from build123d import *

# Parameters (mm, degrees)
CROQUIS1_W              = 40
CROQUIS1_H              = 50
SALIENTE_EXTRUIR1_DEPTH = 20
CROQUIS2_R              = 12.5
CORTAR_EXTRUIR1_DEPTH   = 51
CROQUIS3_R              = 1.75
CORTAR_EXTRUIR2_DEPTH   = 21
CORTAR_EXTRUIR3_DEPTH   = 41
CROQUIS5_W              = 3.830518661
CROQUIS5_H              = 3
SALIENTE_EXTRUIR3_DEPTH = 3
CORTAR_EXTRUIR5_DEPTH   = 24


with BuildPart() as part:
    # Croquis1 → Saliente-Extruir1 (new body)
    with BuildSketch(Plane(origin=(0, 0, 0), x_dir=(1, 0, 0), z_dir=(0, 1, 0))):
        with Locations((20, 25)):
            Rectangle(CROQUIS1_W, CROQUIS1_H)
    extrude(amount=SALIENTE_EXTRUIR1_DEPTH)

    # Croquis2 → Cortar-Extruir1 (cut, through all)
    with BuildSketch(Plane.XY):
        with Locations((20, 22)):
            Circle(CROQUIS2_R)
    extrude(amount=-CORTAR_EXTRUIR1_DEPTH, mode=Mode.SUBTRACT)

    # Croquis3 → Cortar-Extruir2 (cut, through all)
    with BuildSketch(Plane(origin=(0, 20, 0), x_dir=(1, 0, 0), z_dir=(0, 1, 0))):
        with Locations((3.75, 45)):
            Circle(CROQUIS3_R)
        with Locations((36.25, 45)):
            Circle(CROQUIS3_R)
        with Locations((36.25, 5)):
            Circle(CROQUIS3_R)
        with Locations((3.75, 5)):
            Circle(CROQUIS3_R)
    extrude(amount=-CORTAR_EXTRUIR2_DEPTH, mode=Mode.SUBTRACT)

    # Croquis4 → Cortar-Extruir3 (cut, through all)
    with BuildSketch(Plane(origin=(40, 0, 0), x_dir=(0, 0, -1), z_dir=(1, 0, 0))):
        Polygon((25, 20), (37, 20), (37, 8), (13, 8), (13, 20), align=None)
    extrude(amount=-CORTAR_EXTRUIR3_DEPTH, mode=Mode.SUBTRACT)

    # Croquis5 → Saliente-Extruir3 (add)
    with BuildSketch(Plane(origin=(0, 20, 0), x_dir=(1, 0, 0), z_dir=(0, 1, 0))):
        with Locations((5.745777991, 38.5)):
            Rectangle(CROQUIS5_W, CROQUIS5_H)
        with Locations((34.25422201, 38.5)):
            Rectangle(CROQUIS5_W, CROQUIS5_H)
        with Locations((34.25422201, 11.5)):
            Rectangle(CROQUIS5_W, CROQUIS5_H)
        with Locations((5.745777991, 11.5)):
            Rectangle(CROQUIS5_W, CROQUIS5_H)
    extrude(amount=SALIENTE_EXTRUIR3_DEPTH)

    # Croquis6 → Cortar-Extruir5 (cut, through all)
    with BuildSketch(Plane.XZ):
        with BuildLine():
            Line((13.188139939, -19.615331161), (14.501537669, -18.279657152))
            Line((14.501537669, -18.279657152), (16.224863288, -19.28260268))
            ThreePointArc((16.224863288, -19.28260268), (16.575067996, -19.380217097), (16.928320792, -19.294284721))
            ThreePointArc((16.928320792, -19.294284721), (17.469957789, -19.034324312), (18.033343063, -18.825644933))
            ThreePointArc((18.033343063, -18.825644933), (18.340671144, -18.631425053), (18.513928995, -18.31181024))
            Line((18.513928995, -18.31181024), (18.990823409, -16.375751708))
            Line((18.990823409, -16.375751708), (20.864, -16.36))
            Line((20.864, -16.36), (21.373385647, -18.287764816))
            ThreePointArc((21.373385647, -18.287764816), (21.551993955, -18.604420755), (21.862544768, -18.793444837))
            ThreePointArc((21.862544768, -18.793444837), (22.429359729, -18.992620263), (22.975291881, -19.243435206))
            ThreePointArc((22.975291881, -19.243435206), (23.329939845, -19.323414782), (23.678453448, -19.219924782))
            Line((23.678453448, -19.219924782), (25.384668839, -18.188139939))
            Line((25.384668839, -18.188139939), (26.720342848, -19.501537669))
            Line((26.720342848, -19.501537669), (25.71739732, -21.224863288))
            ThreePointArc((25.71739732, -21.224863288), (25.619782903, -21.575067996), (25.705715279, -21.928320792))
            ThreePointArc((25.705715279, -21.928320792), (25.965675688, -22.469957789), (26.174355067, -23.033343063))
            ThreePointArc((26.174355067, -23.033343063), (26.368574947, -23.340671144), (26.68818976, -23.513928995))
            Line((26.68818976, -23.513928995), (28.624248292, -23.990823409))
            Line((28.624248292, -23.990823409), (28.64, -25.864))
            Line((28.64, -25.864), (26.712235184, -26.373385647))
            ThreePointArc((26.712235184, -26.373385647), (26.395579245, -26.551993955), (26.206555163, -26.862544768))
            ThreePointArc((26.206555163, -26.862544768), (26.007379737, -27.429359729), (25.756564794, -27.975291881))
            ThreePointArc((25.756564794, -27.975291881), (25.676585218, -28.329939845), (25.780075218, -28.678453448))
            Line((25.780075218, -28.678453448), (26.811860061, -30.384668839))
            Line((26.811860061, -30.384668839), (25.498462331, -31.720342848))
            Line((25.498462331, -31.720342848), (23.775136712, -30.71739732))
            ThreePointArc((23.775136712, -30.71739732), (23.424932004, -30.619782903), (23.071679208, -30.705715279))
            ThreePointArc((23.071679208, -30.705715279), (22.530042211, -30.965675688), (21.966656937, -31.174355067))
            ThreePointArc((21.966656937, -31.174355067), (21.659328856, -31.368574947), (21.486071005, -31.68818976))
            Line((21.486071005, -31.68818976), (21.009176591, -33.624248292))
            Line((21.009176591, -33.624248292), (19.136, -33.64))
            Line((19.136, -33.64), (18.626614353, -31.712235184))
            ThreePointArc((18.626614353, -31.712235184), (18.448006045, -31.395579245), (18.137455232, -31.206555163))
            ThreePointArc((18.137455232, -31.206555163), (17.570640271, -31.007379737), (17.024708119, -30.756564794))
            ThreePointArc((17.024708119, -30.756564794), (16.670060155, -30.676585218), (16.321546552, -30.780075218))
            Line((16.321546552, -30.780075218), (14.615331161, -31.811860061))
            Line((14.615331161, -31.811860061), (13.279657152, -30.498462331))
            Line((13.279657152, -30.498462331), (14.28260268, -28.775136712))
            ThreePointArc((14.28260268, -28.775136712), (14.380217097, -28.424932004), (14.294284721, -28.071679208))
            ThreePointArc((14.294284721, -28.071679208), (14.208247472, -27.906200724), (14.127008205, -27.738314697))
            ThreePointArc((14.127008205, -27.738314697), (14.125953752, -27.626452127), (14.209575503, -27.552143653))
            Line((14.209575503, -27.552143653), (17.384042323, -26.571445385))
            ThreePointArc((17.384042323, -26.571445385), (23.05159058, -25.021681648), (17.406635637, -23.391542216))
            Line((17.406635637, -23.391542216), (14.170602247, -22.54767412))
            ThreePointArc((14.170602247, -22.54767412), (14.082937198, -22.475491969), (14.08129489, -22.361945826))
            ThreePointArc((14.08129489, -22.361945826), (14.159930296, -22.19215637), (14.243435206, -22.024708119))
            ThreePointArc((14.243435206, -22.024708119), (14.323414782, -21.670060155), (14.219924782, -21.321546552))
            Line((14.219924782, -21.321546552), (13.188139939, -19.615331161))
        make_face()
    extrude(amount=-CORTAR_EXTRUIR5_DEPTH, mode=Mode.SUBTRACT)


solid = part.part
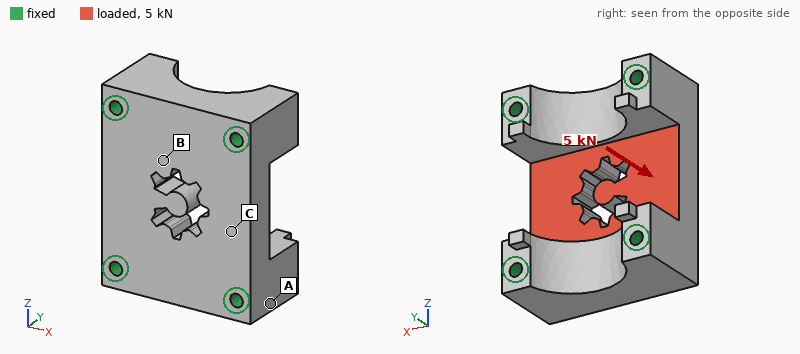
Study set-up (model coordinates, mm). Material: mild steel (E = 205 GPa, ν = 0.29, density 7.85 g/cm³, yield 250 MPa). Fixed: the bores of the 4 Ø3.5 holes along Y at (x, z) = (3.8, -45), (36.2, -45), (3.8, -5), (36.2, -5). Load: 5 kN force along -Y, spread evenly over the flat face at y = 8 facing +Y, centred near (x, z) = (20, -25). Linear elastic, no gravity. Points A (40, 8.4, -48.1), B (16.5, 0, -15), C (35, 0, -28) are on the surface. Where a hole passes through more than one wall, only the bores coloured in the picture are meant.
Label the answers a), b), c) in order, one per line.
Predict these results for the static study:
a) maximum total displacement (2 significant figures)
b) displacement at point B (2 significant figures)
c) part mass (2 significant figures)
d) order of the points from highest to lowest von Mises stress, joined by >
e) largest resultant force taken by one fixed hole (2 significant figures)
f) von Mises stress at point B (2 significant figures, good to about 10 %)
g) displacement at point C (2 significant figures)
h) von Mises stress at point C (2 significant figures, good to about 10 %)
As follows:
a) 10.0 µm
b) 2.8 µm
c) 170 g
d) C > B > A
e) 1.3 kN
f) 10.0 MPa
g) 3.2 µm
h) 26 MPa
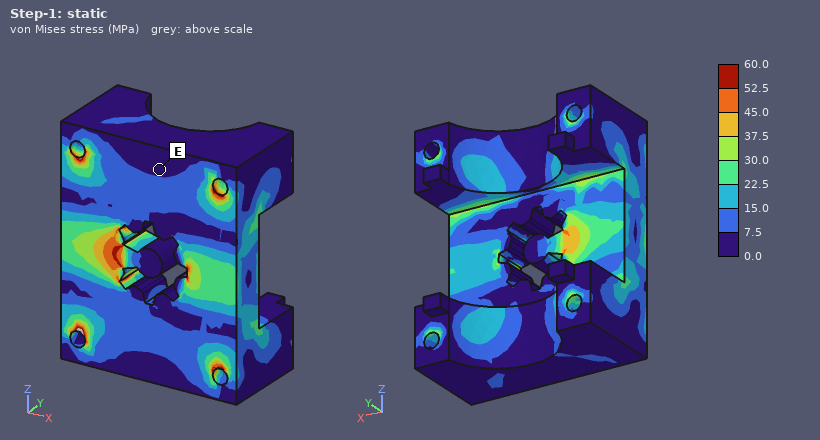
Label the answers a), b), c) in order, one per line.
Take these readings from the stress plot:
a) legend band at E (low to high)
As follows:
a) 0.0 to 7.5 MPa
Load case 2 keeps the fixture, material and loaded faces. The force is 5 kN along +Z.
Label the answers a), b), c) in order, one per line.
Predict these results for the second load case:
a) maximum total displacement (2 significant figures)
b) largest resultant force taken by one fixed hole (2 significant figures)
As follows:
a) 7.1 µm
b) 1.4 kN
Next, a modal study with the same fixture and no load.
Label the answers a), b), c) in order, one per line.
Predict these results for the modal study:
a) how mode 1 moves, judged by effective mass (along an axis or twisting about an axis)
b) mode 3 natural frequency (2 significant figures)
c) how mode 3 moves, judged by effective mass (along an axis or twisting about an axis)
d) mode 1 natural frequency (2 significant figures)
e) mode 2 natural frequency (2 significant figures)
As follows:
a) along Y
b) 30 kHz
c) along Y
d) 22 kHz
e) 27 kHz
